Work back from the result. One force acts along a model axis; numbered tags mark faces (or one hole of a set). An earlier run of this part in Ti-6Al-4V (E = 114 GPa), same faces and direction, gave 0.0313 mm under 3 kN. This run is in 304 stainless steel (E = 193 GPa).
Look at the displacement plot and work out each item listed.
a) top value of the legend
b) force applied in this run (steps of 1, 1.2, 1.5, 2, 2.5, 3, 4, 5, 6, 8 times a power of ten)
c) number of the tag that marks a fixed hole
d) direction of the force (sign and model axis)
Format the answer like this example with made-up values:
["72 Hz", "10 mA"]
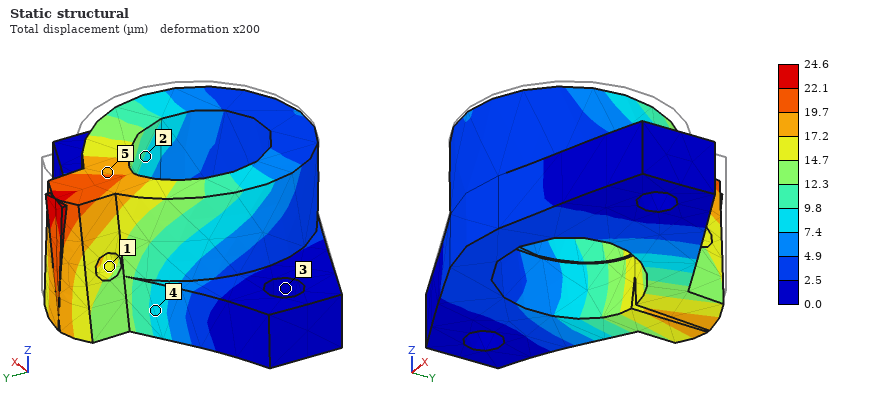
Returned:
["24.6 µm", "4 kN", "3", "-Z"]
